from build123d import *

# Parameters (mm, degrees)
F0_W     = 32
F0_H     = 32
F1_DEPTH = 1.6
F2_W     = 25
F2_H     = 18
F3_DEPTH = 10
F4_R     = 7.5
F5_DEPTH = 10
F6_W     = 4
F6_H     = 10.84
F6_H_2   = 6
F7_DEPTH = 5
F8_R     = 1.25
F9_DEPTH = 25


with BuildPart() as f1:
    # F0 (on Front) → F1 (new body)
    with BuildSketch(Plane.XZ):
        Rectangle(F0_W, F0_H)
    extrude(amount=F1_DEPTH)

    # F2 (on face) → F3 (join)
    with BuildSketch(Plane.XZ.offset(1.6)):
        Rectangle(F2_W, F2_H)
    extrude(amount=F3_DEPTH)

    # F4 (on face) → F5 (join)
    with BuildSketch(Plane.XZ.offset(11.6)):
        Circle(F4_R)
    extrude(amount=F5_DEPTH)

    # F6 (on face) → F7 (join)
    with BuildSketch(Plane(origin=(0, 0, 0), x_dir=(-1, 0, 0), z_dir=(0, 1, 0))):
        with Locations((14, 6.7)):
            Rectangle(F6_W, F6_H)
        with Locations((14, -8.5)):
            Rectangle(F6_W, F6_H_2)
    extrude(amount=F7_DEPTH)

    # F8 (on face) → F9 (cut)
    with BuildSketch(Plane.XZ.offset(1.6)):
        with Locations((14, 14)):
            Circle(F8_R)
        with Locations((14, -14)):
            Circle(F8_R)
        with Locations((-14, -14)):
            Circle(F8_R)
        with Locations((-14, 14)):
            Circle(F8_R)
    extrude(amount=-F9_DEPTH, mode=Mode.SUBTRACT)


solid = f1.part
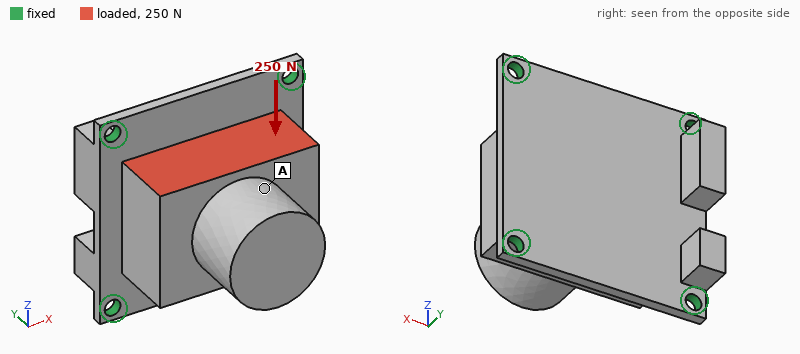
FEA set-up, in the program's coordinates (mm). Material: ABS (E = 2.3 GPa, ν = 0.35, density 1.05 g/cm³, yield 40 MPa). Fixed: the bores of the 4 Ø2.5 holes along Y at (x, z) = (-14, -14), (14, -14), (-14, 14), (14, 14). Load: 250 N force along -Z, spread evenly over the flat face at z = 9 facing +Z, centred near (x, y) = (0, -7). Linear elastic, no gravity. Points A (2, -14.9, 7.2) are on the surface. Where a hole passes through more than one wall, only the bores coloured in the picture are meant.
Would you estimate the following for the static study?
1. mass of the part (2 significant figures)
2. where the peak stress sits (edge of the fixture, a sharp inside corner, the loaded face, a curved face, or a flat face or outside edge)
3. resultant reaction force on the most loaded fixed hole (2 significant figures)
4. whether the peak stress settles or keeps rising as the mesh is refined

8.6 g
edge of the fixture
79 N
keeps rising
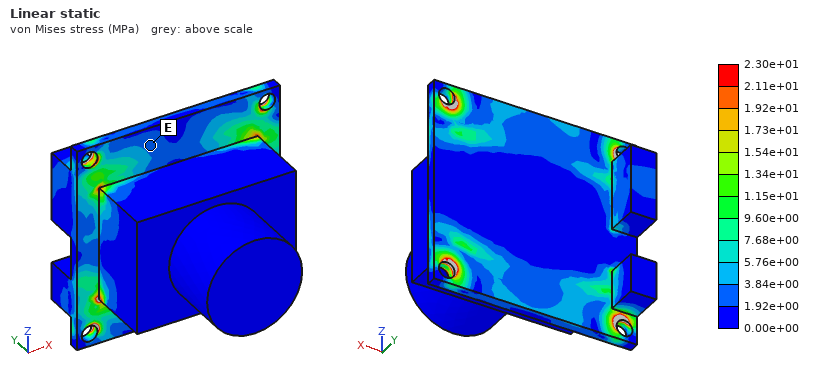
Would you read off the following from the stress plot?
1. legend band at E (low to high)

1.92e+00 to 3.84e+00 MPa
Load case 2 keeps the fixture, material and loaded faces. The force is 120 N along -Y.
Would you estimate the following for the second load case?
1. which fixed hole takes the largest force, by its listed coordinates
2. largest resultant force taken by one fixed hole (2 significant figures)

(-14, 14)
59 N
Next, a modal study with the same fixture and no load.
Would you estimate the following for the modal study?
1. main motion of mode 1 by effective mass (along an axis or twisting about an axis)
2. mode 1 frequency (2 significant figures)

along Y
1900 Hz
